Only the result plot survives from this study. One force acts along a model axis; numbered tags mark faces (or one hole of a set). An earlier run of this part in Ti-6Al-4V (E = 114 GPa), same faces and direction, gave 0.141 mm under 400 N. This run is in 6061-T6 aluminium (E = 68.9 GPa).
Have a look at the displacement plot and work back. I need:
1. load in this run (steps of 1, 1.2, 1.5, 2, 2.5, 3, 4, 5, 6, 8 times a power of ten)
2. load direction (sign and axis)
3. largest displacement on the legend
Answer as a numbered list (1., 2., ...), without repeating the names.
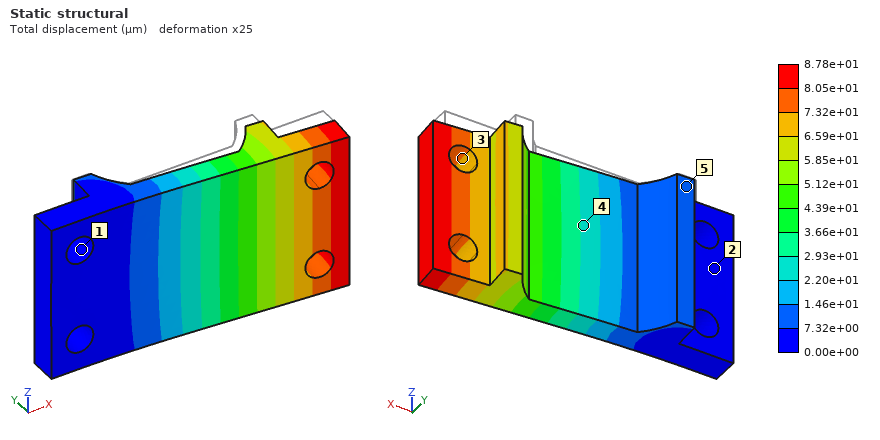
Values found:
1. 150 N
2. -Y
3. 8.78e+01 µm
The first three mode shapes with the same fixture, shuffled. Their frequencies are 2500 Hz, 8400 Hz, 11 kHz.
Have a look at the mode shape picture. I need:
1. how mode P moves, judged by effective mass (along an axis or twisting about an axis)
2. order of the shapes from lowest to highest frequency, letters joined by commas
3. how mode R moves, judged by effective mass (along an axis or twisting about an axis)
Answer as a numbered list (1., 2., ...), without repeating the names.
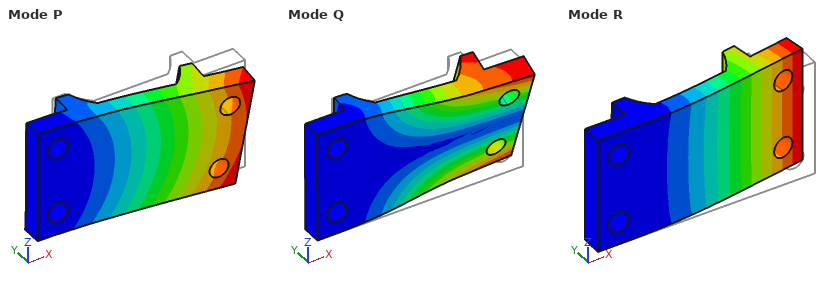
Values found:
1. along Z
2. R, Q, P
3. along Y
